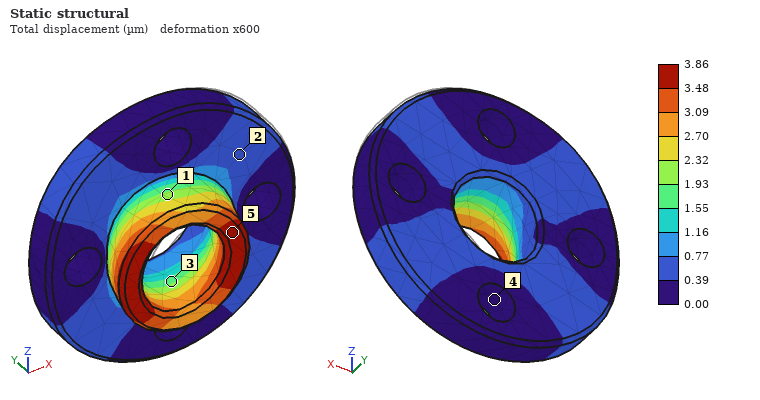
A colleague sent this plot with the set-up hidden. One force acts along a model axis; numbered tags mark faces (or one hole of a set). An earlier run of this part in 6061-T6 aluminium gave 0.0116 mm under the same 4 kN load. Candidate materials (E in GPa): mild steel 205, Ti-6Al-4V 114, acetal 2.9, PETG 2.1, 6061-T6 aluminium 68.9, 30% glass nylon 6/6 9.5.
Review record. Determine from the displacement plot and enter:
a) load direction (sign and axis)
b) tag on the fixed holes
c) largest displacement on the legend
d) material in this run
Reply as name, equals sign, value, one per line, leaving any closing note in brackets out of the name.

load direction = -X
tag on the fixed holes = 4
largest displacement on the legend = 3.86 µm
material in this run = mild steel
